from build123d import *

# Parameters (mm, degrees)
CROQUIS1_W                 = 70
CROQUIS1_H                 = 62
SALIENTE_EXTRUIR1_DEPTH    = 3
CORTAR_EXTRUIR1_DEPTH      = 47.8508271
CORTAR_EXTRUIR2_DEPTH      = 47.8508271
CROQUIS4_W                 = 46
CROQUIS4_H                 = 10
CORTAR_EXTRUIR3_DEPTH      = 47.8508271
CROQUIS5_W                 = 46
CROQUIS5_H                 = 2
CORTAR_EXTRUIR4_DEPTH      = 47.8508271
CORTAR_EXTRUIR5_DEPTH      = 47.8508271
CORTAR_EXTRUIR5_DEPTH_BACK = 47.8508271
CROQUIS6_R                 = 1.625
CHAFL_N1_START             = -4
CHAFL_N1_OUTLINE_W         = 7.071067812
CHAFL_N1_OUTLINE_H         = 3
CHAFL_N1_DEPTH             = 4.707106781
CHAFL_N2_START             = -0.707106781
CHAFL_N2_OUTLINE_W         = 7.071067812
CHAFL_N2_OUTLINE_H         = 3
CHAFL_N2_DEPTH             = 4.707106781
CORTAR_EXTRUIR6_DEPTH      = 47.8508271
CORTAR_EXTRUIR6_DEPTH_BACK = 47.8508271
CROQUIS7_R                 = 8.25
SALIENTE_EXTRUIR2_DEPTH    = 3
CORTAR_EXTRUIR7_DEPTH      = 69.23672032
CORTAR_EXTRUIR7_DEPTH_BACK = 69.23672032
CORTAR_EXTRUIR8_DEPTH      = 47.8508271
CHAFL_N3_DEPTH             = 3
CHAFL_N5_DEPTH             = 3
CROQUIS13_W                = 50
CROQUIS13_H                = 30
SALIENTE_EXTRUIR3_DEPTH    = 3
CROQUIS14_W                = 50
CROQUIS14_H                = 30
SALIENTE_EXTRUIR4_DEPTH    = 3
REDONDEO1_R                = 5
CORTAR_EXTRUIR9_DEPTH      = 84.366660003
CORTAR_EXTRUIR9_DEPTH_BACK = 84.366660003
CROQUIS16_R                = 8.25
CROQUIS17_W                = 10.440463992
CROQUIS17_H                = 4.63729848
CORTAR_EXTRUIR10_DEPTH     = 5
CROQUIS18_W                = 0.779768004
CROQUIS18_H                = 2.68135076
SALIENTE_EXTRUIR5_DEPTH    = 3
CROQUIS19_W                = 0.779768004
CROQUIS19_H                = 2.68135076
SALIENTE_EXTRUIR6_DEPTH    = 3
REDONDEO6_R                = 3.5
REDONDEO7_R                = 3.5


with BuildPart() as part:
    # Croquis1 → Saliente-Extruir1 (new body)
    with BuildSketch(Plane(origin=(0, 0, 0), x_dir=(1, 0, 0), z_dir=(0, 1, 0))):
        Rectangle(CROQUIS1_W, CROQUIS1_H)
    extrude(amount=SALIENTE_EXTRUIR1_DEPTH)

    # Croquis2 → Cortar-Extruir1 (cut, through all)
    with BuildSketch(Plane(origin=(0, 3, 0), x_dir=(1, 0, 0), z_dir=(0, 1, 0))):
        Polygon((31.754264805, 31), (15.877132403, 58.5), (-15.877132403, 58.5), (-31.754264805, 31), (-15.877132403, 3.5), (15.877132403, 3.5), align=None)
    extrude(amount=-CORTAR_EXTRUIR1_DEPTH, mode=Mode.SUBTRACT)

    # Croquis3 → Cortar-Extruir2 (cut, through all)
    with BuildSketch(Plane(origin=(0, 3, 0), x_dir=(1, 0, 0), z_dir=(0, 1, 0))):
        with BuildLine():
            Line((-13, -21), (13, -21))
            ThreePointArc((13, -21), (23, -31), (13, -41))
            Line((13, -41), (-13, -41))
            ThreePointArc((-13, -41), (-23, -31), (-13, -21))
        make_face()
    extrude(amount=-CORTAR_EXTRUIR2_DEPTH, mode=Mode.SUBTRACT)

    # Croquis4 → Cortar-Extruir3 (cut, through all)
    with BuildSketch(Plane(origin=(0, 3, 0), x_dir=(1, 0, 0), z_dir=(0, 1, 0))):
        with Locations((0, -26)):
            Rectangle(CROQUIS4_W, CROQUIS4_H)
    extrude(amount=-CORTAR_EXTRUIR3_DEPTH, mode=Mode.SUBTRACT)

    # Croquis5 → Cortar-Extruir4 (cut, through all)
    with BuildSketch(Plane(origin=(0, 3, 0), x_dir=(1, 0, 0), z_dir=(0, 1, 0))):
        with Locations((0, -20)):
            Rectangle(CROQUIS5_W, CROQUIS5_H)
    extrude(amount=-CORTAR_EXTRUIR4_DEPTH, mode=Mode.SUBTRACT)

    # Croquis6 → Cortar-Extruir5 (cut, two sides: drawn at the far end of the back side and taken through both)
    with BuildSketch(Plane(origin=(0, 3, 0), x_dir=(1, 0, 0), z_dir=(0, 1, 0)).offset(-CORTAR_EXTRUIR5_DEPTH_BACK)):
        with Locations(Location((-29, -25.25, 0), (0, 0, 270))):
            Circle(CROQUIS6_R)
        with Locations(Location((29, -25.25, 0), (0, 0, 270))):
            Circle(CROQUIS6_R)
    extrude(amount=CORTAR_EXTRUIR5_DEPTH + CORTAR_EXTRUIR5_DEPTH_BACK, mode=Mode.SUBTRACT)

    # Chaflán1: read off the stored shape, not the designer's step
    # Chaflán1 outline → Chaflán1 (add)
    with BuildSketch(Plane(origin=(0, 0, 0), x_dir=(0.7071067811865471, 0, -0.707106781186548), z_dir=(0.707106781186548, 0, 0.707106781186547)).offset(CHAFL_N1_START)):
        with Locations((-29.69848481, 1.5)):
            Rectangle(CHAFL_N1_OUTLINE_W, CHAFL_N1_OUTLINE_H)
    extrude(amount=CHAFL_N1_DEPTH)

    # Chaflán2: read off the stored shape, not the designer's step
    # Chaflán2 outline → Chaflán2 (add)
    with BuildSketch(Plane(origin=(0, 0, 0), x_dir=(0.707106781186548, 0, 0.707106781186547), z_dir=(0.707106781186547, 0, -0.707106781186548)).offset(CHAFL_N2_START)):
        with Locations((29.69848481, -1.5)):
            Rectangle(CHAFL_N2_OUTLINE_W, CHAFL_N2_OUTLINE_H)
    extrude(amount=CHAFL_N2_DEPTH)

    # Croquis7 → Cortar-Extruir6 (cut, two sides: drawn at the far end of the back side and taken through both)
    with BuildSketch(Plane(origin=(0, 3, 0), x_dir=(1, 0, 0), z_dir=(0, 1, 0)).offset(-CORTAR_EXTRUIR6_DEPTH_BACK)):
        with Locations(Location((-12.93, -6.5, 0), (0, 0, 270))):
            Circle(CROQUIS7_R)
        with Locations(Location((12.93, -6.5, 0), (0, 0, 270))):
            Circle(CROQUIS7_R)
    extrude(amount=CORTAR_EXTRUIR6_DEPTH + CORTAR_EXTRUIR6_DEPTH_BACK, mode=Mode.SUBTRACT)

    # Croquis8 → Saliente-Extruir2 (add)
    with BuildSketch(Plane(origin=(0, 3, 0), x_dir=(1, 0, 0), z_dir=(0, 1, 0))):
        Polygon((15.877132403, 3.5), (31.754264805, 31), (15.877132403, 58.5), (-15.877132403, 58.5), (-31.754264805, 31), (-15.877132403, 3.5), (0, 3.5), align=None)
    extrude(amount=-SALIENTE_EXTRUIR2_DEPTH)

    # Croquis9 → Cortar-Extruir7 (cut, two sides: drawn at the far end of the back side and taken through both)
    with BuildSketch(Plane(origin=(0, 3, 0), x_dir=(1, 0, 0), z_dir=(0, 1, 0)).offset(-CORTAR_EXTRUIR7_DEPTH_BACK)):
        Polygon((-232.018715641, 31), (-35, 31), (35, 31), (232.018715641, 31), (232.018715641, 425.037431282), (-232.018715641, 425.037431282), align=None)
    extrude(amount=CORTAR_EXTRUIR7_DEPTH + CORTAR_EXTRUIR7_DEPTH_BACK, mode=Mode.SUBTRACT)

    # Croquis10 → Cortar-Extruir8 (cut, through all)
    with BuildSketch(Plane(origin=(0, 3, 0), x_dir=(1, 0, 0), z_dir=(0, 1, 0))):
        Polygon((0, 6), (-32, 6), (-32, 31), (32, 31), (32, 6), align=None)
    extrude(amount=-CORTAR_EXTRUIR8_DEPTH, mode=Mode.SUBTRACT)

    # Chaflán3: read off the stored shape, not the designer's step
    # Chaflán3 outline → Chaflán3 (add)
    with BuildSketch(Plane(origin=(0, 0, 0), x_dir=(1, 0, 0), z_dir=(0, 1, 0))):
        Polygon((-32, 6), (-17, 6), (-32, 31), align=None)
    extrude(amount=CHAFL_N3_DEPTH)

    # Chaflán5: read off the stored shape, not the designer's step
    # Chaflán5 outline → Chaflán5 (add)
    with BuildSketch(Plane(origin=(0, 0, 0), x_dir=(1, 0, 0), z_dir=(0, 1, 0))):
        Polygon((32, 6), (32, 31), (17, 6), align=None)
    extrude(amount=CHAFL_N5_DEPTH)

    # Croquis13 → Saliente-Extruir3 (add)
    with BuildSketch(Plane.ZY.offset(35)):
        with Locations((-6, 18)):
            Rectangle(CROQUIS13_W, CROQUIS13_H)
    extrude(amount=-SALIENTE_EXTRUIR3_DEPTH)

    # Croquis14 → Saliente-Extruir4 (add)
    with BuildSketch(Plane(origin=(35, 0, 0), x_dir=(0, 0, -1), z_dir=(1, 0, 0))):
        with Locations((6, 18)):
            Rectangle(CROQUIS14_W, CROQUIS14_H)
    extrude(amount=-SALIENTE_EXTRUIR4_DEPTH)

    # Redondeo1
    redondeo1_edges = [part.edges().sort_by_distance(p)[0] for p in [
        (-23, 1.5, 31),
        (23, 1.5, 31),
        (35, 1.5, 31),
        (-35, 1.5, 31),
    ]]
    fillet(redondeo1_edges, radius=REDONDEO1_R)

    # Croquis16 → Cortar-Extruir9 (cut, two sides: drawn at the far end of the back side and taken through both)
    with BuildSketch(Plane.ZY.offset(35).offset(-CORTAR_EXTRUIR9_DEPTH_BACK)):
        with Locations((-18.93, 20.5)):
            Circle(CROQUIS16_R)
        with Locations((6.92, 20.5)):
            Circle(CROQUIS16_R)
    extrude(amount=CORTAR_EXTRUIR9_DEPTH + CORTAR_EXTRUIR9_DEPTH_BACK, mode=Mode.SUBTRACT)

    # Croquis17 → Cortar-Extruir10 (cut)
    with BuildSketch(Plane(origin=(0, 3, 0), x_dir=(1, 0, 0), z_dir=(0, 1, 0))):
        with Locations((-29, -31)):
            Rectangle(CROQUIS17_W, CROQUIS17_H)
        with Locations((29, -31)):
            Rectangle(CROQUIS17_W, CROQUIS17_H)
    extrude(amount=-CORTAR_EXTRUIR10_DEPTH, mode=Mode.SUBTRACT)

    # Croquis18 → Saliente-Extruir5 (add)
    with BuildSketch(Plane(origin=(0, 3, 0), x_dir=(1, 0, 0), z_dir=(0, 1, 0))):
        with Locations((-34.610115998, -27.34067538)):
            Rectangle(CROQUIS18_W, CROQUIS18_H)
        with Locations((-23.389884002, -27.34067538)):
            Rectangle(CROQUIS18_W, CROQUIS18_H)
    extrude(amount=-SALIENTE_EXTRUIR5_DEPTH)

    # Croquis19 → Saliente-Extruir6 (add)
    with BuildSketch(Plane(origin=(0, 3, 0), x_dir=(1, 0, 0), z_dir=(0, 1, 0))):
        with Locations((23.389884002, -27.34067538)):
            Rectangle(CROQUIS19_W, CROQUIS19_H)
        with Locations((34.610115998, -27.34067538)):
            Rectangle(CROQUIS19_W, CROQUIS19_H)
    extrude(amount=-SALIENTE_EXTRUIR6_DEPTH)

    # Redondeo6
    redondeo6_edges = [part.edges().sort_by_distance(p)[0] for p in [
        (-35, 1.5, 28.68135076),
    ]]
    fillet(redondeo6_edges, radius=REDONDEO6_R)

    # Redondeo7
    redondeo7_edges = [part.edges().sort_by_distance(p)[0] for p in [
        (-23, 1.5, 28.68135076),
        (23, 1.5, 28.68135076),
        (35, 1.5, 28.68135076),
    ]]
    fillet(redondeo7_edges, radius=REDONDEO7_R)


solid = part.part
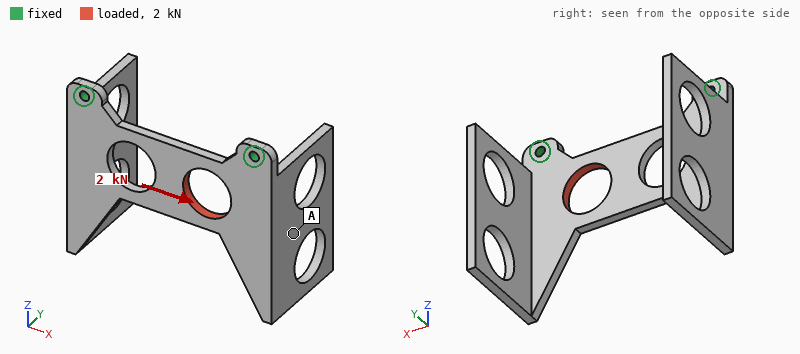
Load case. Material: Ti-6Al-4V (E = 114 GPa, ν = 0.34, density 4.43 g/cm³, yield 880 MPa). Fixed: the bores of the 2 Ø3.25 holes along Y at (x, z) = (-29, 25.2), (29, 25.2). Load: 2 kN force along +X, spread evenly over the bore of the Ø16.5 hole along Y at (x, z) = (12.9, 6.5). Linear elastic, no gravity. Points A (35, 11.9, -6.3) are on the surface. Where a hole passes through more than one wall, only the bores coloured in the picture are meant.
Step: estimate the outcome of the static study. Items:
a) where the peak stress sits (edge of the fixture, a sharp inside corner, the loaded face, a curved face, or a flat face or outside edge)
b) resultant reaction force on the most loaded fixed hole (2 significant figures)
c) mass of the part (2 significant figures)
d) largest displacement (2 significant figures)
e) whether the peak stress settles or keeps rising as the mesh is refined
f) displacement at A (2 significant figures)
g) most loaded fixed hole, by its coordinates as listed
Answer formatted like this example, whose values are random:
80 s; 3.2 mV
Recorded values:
edge of the fixture; 1.2 kN; 56 g; 60 µm; keeps rising; 39 µm; (29, 25.2)
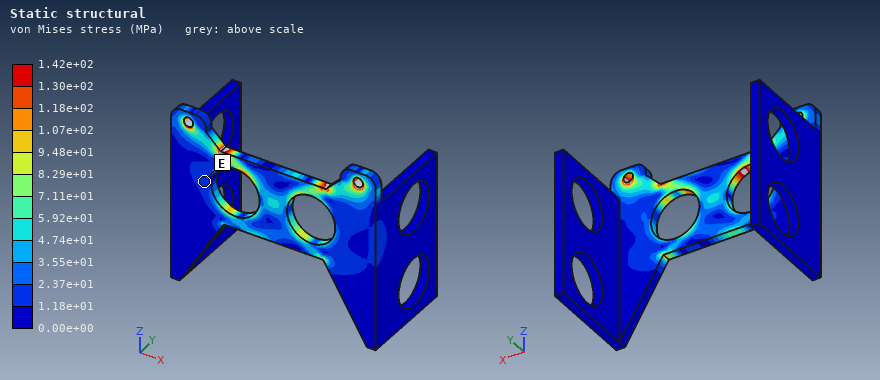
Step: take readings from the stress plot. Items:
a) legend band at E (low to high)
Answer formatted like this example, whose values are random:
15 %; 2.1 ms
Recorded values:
1.18e+01 to 2.37e+01 MPa
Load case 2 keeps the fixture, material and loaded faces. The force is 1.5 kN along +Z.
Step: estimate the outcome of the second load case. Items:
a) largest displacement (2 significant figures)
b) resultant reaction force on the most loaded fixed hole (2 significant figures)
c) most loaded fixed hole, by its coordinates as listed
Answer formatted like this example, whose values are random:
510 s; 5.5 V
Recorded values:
25 µm; 1.2 kN; (29, 25.2)
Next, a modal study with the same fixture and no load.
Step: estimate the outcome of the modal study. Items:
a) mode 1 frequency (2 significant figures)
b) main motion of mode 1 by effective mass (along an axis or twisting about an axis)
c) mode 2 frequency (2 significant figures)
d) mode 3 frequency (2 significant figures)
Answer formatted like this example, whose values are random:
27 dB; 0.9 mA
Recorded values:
610 Hz; along Y; 720 Hz; 1200 Hz
